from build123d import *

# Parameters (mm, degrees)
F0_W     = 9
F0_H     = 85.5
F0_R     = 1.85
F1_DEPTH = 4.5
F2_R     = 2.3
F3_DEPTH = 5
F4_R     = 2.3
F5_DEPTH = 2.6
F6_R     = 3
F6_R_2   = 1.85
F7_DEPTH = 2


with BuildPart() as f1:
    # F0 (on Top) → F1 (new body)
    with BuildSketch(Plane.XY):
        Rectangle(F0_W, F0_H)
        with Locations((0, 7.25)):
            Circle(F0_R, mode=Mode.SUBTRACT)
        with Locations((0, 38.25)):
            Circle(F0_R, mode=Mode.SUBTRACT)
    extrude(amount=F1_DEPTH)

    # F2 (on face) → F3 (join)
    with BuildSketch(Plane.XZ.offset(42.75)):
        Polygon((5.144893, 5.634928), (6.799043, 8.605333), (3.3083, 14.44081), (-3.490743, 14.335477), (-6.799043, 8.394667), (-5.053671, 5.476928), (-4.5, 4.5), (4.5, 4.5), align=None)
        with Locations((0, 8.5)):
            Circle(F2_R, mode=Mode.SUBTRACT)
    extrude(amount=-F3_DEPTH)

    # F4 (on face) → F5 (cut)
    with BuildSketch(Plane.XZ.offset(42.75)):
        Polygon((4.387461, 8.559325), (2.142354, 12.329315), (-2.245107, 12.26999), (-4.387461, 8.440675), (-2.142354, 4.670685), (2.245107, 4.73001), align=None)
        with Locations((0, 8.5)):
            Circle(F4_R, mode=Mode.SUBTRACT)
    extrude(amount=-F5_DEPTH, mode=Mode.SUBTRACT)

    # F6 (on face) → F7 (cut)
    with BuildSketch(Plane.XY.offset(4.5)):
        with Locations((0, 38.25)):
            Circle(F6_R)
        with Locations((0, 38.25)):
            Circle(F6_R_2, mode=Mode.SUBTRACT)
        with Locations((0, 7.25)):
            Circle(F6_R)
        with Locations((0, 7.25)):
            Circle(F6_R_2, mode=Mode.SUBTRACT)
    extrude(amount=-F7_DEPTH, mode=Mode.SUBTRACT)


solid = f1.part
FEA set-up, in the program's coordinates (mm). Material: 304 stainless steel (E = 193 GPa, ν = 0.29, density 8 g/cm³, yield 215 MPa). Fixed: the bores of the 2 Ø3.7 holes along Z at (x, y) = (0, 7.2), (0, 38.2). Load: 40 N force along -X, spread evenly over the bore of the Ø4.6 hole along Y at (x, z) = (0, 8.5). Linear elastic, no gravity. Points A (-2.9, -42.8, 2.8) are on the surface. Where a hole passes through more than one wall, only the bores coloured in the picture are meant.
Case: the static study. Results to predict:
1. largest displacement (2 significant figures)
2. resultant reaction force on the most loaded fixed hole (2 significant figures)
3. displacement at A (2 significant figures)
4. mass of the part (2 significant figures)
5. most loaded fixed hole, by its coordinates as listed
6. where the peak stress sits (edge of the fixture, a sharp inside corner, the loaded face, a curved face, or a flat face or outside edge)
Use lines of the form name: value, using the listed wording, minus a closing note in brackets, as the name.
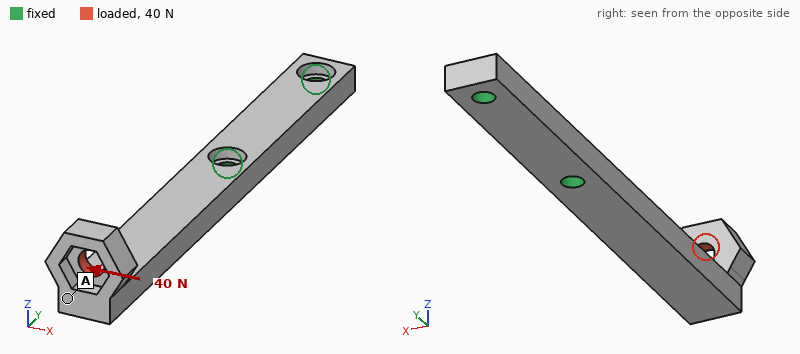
largest displacement: 45 µm
resultant reaction force on the most loaded fixed hole: 64 N
displacement at A: 35 µm
mass of the part: 29 g
most loaded fixed hole, by its coordinates as listed: (0, 7.2)
where the peak stress sits: edge of the fixture
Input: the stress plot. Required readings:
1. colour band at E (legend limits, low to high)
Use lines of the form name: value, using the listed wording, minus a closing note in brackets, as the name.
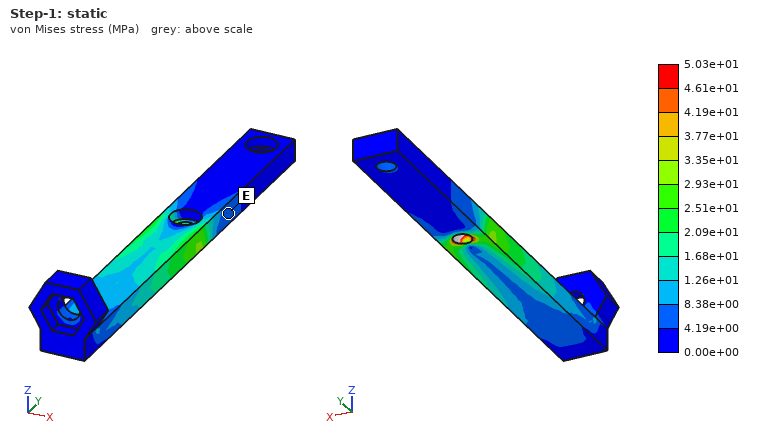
colour band at E: 4.19e+00 to 8.38e+00 MPa
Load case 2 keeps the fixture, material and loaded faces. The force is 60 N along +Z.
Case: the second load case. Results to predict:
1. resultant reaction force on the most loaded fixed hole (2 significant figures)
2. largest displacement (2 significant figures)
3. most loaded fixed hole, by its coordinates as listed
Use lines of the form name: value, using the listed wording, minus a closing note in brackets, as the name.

resultant reaction force on the most loaded fixed hole: 120 N
largest displacement: 0.21 mm
most loaded fixed hole, by its coordinates as listed: (0, 7.2)
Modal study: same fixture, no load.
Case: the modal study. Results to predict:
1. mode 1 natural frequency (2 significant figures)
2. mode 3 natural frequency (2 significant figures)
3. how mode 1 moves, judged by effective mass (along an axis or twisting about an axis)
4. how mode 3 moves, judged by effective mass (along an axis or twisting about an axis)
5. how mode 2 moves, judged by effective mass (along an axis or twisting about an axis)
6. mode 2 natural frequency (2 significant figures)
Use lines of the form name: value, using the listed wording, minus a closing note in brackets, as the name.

mode 1 natural frequency: 1000 Hz
mode 3 natural frequency: 5800 Hz
how mode 1 moves, judged by effective mass: along Z
how mode 3 moves, judged by effective mass: twisting about Y
how mode 2 moves, judged by effective mass: along X
mode 2 natural frequency: 2000 Hz
